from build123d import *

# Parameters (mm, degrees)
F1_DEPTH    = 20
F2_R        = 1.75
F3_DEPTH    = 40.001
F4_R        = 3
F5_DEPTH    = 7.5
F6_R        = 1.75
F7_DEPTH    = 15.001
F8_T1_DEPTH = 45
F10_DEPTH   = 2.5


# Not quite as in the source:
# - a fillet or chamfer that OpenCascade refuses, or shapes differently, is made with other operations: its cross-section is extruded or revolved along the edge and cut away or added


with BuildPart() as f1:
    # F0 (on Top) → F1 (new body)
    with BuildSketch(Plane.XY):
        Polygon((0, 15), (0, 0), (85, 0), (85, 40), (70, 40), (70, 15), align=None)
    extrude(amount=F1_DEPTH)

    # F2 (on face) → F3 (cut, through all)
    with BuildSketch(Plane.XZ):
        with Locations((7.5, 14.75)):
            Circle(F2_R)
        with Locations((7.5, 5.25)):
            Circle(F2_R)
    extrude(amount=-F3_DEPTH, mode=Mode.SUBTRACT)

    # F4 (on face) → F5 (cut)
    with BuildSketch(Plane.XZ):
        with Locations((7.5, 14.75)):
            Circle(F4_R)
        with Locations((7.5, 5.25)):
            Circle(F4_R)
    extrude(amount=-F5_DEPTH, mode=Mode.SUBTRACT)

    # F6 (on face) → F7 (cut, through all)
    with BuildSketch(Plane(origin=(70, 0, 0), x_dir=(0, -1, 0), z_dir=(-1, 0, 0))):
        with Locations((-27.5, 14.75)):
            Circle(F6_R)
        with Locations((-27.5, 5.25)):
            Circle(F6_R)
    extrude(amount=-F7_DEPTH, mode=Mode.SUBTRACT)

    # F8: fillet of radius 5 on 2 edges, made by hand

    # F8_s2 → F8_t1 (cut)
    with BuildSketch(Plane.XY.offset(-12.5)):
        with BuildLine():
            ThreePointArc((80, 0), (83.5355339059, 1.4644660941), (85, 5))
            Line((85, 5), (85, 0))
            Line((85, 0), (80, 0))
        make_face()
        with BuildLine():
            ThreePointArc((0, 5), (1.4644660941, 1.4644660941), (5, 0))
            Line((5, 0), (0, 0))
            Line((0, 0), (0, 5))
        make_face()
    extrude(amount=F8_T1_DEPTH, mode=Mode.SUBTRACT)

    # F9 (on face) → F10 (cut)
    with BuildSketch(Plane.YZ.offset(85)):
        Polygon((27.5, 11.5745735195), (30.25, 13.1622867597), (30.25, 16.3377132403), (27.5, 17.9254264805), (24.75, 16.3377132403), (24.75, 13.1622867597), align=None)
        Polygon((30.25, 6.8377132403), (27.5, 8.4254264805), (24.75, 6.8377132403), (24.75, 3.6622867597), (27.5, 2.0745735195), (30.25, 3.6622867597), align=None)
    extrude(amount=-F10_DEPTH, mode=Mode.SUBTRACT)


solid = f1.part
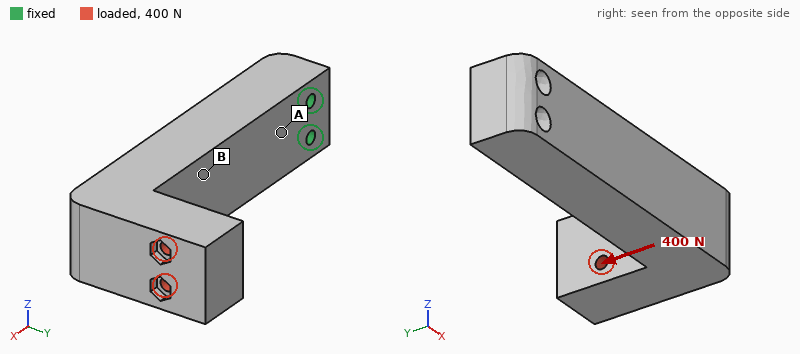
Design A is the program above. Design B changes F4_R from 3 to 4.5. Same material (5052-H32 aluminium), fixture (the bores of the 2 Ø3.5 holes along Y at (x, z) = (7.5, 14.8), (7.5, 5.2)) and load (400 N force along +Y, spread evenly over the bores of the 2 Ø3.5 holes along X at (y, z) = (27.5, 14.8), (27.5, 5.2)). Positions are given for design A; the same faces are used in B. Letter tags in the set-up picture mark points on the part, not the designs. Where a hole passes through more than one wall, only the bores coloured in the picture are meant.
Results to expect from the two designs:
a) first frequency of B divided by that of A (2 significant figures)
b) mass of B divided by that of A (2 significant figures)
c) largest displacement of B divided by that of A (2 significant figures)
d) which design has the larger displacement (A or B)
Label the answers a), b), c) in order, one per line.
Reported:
a) 0.92
b) 0.98
c) 1.2
d) B
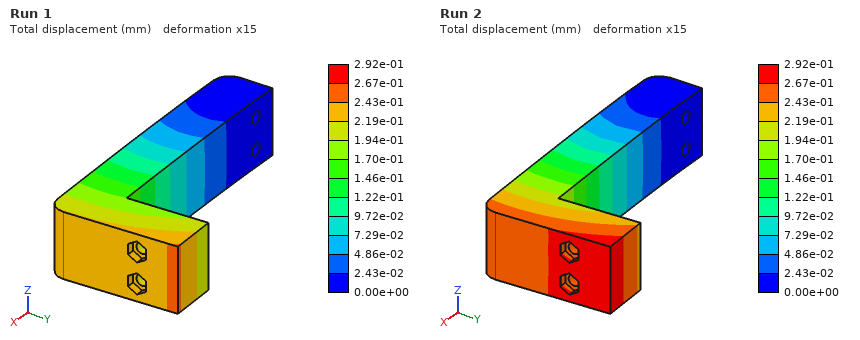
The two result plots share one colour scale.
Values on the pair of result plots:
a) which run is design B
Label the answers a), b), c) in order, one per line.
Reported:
a) Run 2
